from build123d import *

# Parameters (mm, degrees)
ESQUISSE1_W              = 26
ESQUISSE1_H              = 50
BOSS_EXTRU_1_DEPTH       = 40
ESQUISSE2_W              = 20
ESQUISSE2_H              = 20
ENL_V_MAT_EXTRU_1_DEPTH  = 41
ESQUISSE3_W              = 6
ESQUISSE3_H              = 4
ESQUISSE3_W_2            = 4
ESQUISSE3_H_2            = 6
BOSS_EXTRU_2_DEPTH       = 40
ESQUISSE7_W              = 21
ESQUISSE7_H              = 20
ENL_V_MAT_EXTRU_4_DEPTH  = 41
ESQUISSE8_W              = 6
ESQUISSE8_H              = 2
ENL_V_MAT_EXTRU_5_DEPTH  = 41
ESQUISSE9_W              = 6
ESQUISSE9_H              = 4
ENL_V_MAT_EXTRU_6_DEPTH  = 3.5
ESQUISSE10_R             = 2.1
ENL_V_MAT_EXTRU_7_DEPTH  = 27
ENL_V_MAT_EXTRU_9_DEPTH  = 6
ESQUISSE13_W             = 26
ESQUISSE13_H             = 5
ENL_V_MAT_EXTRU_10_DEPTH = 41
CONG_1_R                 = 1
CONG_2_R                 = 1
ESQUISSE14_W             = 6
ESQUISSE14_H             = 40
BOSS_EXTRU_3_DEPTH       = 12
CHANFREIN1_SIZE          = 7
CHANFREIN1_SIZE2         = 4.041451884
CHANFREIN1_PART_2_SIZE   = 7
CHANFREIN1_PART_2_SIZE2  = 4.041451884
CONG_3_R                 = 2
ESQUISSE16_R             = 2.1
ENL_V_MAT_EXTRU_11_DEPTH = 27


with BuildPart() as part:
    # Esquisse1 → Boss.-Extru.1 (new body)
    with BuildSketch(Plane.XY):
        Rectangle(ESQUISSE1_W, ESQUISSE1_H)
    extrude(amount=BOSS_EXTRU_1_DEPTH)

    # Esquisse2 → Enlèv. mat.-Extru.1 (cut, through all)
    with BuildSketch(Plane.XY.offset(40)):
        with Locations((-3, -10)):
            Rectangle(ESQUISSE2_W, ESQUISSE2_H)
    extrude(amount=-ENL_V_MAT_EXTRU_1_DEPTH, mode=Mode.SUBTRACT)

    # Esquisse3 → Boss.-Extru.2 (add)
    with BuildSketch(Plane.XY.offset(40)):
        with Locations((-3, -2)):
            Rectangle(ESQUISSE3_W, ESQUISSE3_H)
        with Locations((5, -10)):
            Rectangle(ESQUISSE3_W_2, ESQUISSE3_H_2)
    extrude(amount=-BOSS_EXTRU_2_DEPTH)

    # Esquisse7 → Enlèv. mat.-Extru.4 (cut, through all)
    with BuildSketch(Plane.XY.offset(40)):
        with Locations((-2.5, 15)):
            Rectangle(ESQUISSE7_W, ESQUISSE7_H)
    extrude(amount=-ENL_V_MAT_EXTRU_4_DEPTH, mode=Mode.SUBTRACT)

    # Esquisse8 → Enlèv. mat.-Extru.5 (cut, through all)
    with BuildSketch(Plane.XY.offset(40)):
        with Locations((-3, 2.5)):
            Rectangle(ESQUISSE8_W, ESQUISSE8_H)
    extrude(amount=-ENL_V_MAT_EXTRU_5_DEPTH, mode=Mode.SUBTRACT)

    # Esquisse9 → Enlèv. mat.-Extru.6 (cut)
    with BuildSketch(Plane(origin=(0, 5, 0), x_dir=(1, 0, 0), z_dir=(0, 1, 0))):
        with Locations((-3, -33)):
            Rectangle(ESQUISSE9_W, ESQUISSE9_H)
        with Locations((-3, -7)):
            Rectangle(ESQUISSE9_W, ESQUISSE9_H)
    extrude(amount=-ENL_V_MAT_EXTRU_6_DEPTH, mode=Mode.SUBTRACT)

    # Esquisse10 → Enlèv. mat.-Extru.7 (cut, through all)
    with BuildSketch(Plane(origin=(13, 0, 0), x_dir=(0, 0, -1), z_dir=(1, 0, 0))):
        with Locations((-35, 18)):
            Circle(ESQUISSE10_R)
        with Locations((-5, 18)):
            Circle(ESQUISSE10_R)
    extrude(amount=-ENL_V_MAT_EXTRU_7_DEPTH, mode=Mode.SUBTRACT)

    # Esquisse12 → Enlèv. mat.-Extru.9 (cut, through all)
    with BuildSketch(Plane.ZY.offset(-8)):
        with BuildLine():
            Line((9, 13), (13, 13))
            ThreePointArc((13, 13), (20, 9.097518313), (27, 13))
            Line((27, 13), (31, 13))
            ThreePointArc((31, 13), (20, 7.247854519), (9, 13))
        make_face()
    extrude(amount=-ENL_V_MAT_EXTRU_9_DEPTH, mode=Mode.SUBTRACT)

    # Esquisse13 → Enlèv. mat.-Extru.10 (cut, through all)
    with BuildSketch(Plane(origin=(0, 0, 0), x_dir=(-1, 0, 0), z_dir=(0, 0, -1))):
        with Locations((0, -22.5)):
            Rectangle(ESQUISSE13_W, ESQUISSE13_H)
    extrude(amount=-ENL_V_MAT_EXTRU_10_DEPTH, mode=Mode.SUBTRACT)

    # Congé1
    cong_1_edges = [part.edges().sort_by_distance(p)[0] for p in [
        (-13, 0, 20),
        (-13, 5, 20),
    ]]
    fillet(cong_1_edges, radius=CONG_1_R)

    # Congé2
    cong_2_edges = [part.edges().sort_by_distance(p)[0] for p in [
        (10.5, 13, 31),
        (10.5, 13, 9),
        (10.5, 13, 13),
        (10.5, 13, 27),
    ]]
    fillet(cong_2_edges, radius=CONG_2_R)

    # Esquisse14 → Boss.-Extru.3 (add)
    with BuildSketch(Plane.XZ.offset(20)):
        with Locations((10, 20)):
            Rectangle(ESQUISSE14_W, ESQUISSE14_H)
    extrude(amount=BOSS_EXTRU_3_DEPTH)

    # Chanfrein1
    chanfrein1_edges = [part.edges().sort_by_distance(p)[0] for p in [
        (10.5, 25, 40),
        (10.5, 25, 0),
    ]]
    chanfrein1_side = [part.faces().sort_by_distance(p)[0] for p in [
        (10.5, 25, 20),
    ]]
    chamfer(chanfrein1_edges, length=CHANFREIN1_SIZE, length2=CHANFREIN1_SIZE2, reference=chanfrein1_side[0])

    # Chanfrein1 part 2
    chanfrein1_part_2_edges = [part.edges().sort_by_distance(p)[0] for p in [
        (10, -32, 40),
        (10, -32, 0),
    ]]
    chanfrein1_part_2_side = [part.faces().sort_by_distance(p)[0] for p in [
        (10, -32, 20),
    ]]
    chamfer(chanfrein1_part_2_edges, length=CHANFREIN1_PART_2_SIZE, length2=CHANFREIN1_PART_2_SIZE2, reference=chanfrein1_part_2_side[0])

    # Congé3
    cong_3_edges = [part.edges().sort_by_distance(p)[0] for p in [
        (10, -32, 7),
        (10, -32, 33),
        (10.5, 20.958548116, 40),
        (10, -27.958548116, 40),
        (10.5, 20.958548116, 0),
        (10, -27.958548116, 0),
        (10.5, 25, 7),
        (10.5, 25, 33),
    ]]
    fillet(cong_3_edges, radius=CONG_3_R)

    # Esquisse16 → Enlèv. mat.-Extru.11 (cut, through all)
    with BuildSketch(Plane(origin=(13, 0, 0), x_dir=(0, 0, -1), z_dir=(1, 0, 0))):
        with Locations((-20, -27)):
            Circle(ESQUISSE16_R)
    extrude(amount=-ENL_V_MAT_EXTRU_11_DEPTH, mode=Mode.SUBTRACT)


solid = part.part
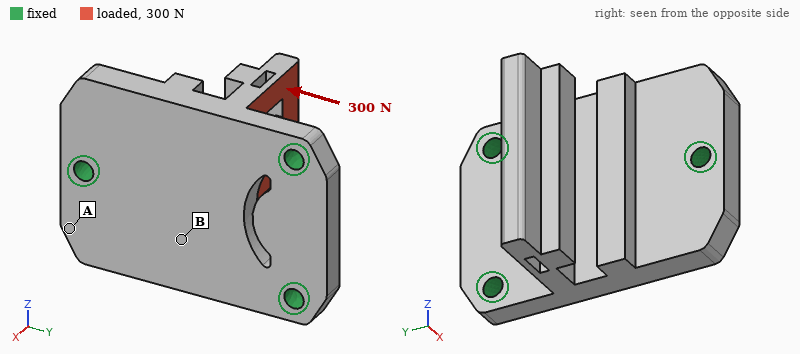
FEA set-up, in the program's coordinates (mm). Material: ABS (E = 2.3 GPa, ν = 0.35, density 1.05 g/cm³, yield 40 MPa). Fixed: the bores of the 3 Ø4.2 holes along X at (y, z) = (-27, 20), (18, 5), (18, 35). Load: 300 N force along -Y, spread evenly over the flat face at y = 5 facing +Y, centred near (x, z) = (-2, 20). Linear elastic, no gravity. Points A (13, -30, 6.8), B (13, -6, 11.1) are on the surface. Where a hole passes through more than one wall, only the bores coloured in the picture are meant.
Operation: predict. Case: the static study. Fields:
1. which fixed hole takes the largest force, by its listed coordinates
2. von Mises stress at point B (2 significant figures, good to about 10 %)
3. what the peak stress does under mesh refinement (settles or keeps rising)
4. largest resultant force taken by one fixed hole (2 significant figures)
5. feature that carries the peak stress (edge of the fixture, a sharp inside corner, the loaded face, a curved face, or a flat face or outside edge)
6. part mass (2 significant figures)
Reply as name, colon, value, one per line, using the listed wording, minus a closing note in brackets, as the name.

which fixed hole takes the largest force, by its listed coordinates: (-27, 20)
von Mises stress at point B: 4.8 MPa
what the peak stress does under mesh refinement: keeps rising
largest resultant force taken by one fixed hole: 190 N
feature that carries the peak stress: edge of the fixture
part mass: 18 g
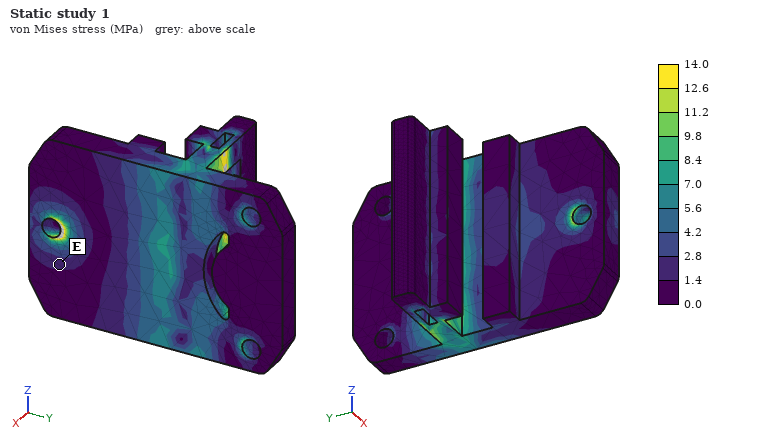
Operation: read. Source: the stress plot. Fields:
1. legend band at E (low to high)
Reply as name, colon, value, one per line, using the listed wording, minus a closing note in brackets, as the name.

legend band at E: 1.4 to 2.8 MPa
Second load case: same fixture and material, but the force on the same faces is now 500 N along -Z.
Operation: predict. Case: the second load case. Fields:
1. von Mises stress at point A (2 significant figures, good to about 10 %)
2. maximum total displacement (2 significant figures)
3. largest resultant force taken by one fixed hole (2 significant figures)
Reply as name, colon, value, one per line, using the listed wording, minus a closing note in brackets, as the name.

von Mises stress at point A: 2.4 MPa
maximum total displacement: 0.57 mm
largest resultant force taken by one fixed hole: 230 N
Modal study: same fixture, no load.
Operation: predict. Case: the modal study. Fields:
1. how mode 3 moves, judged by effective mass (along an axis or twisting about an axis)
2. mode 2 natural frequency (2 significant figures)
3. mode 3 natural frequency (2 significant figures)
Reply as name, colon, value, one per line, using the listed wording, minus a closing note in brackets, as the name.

how mode 3 moves, judged by effective mass: along X
mode 2 natural frequency: 2000 Hz
mode 3 natural frequency: 2500 Hz
